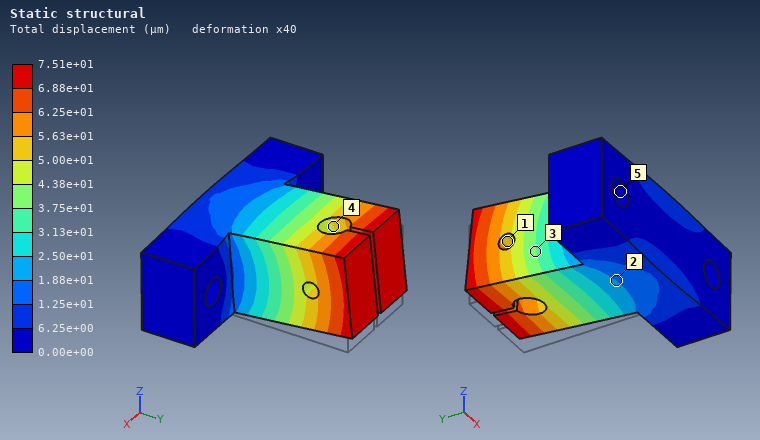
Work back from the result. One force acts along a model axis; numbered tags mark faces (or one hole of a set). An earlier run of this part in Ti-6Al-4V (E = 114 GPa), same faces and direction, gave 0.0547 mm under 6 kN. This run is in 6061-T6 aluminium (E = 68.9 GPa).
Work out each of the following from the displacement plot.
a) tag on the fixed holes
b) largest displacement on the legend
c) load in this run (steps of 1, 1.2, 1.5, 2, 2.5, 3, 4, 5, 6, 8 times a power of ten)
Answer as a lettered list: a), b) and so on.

a) 5
b) 7.51e+01 µm
c) 5 kN
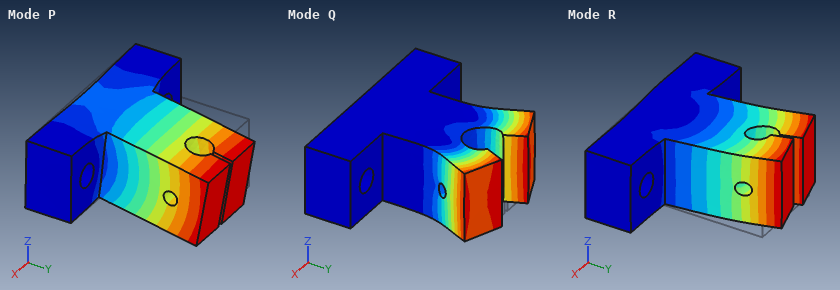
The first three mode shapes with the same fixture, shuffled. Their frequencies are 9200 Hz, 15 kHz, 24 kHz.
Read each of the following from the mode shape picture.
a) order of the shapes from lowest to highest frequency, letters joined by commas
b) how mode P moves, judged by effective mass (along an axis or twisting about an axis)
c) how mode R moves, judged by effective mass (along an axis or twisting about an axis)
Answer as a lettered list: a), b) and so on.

a) P, R, Q
b) along Z
c) along X
